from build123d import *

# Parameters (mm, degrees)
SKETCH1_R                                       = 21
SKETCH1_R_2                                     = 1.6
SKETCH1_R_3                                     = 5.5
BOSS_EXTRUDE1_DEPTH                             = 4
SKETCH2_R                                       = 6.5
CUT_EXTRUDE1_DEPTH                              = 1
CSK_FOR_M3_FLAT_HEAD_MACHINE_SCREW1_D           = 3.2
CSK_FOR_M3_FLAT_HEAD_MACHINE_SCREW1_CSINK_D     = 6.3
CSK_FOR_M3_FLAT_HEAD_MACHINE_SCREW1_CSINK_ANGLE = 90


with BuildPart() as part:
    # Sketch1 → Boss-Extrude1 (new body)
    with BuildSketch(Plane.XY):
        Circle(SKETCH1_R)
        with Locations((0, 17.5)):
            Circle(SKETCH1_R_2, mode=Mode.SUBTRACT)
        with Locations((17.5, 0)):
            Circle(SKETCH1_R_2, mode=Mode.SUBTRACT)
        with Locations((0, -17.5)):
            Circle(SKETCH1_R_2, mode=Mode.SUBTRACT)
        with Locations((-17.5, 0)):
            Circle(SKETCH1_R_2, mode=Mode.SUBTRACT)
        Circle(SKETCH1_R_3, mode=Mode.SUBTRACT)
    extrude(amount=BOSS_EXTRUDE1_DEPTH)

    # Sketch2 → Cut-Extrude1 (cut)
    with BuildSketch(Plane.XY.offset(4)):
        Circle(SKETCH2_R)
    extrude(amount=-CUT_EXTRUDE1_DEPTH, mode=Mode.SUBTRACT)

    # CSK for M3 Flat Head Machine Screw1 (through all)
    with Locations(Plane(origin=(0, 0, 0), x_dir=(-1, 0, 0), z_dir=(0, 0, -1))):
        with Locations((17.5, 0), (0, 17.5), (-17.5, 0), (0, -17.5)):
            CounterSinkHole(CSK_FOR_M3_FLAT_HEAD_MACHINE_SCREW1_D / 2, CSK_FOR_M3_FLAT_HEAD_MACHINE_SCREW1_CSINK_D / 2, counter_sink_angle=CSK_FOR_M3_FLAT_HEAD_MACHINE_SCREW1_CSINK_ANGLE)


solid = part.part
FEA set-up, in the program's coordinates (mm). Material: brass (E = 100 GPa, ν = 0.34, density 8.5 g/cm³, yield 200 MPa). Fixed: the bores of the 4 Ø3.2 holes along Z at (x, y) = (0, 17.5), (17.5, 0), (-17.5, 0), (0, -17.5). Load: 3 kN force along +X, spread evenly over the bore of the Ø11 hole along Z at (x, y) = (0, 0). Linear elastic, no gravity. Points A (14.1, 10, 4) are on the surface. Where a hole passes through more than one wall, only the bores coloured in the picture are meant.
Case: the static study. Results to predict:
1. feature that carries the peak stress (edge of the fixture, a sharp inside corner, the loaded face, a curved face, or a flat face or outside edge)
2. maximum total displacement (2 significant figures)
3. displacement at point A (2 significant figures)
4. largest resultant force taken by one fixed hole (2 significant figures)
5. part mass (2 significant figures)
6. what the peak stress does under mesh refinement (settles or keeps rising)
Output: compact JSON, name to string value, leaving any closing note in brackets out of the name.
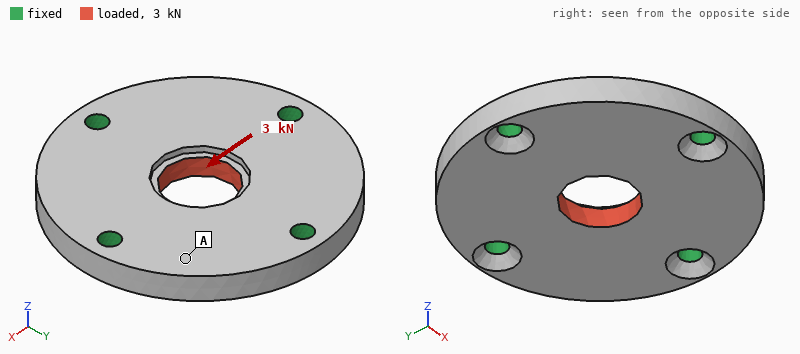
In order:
{"feature that carries the peak stress": "edge of the fixture", "maximum total displacement": "4.3 µm", "displacement at point A": "2.0 µm", "largest resultant force taken by one fixed hole": "950 N", "part mass": "42 g", "what the peak stress does under mesh refinement": "keeps rising"}
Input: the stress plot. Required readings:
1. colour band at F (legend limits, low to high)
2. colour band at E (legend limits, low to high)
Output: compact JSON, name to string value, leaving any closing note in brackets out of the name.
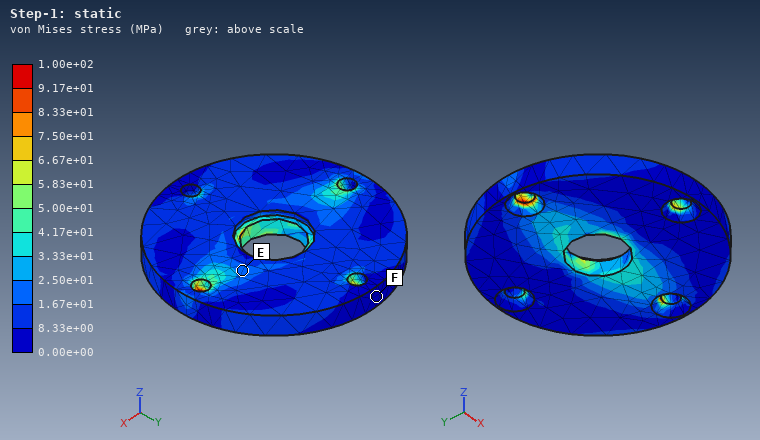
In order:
{"colour band at F": "0.00e+00 to 8.33e+00 MPa", "colour band at E": "1.67e+01 to 2.50e+01 MPa"}
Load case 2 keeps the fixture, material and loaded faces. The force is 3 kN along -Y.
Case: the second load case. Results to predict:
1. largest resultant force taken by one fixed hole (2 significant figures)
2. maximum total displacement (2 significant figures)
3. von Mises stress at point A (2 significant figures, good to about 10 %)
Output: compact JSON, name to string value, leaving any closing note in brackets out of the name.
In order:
{"largest resultant force taken by one fixed hole": "950 N", "maximum total displacement": "4.3 µm", "von Mises stress at point A": "8.8 MPa"}
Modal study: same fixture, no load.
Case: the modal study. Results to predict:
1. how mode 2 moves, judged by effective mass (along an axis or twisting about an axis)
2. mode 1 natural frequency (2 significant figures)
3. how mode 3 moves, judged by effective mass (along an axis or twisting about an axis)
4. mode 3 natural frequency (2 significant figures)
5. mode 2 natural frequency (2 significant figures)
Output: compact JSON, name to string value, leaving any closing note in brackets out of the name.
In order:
{"how mode 2 moves, judged by effective mass": "along Z", "mode 1 natural frequency": "14 kHz", "how mode 3 moves, judged by effective mass": "twisting about X", "mode 3 natural frequency": "15 kHz", "mode 2 natural frequency": "15 kHz"}
